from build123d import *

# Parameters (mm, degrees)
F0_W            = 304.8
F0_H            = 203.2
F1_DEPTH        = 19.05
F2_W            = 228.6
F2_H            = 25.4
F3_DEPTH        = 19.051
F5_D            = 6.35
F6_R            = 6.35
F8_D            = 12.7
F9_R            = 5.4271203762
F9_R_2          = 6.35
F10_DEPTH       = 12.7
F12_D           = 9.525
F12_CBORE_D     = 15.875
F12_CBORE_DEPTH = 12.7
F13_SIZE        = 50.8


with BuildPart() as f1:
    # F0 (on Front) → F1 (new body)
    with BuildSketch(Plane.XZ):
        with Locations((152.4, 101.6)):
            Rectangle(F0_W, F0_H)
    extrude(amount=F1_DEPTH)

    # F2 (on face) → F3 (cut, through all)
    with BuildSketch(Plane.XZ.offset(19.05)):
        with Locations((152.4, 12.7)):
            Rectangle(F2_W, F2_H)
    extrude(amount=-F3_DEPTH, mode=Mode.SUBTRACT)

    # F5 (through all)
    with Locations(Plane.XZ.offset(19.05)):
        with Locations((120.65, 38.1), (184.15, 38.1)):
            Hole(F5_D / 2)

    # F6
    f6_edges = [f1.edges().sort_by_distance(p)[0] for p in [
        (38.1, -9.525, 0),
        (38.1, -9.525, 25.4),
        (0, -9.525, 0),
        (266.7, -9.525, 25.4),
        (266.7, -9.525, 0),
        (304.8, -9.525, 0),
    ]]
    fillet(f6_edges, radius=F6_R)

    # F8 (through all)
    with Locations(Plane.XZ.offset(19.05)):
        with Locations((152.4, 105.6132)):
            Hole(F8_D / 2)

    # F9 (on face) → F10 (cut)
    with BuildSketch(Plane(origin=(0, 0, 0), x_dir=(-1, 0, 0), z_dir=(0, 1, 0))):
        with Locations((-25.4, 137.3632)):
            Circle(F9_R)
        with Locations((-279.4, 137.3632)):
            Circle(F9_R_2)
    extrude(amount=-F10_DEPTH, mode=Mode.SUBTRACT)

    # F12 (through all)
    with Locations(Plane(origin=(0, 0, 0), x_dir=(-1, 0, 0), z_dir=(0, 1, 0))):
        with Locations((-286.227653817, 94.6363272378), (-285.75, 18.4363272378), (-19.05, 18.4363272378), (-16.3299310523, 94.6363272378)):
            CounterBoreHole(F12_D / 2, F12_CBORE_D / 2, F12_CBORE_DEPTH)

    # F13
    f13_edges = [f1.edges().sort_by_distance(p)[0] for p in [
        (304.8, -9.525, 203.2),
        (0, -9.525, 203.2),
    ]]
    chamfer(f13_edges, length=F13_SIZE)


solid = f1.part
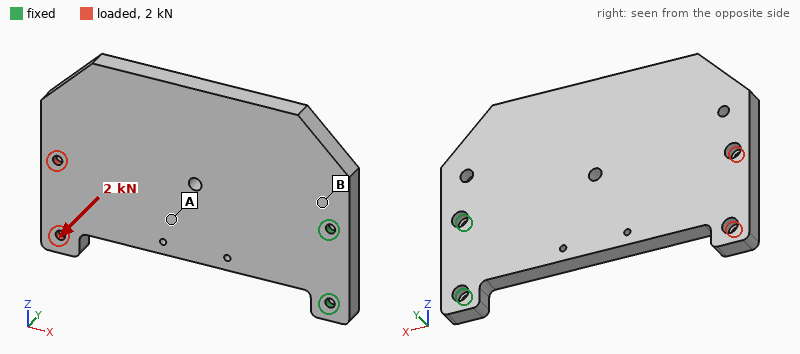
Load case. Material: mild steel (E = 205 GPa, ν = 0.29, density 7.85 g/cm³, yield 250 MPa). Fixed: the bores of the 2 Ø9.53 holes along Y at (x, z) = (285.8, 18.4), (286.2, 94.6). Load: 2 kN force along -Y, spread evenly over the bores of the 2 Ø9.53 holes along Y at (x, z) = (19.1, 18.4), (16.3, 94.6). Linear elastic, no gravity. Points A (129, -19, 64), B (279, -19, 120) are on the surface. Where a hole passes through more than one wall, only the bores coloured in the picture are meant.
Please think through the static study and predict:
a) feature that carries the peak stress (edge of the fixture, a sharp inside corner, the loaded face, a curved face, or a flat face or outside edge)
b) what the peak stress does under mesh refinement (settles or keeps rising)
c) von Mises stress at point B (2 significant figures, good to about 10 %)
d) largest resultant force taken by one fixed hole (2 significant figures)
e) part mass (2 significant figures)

edge of the fixture
keeps rising
60 MPa
2.7 kN
7.9 kg
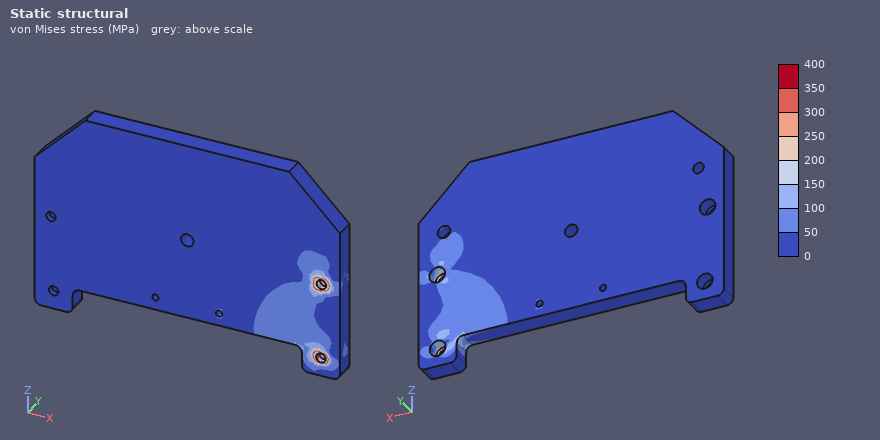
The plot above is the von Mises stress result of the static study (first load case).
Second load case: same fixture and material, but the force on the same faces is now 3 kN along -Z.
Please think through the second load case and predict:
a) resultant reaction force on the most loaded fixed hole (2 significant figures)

11 kN
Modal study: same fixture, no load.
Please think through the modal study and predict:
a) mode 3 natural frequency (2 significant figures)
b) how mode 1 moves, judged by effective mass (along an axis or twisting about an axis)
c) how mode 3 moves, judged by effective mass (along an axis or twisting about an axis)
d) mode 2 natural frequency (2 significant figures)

600 Hz
along Y
along Z
460 Hz
